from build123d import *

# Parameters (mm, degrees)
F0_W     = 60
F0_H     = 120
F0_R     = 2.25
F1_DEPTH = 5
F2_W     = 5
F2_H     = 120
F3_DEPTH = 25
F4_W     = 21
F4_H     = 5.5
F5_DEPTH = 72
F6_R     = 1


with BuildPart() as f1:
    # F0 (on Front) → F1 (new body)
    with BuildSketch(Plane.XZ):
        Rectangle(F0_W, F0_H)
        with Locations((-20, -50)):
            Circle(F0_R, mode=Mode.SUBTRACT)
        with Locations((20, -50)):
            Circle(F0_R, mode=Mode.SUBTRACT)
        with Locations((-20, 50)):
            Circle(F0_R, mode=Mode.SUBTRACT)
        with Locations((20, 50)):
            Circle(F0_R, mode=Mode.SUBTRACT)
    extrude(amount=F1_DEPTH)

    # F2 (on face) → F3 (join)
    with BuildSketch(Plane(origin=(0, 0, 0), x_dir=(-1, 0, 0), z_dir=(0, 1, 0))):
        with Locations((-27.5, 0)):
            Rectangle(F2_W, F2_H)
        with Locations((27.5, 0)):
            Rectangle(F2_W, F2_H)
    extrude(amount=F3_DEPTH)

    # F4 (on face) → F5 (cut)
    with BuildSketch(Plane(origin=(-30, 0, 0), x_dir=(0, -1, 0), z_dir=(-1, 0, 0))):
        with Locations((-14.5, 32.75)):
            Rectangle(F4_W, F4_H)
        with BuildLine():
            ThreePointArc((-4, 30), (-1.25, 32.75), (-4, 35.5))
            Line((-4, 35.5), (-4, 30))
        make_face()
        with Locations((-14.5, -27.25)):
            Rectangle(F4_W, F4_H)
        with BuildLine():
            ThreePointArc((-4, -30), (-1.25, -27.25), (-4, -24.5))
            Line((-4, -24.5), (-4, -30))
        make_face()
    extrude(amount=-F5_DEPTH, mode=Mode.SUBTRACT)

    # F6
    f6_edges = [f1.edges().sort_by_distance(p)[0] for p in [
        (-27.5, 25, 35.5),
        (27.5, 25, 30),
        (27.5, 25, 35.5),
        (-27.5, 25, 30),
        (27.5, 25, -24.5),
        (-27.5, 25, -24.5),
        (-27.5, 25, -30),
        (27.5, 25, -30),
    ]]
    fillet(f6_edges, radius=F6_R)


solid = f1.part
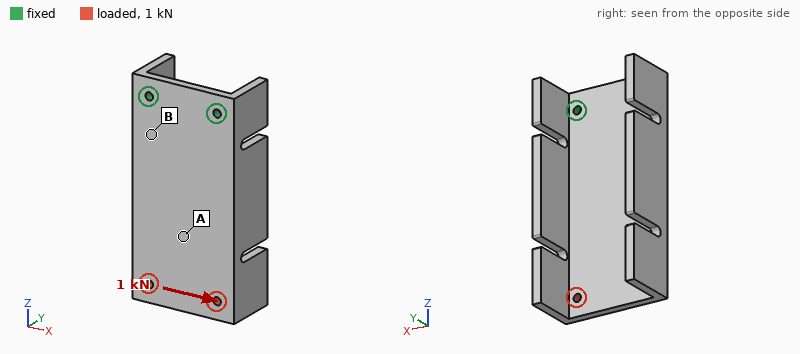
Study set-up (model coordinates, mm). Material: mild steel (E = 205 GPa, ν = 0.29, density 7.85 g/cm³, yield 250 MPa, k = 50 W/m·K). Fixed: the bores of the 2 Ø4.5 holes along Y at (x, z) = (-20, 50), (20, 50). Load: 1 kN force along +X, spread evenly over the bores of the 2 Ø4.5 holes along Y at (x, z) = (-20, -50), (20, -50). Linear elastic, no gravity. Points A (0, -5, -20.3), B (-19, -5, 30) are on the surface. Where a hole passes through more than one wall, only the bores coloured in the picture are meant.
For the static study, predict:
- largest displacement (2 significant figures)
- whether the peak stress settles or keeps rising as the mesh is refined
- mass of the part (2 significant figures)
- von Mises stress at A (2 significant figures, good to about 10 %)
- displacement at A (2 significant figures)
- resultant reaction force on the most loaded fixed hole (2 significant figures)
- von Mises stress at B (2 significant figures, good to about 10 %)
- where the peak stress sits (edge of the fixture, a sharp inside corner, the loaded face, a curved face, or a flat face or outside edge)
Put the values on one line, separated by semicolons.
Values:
29 µm; keeps rising; 500 g; 5.5 MPa; 14 µm; 2.4 kN; 16 MPa; edge of the fixture
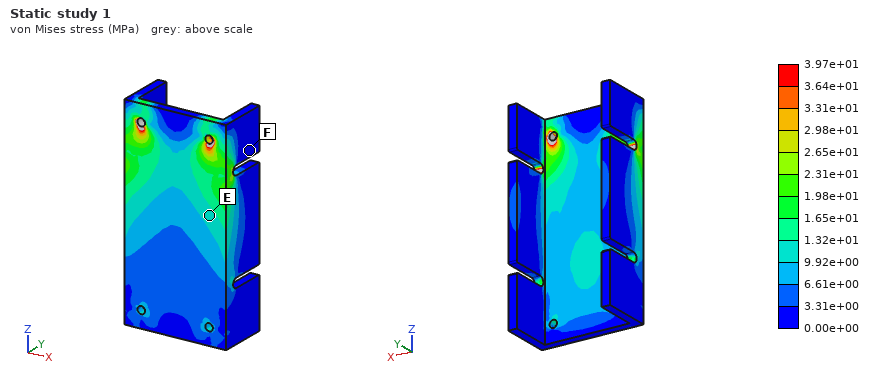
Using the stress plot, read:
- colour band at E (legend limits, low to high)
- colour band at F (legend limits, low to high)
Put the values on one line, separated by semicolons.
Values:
9.92e+00 to 1.32e+01 MPa; 0.00e+00 to 3.31e+00 MPa
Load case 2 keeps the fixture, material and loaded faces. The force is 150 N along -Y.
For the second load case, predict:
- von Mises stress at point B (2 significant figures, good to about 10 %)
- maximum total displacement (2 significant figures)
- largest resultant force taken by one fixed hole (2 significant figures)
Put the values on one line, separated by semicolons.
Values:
33 MPa; 0.21 mm; 110 N
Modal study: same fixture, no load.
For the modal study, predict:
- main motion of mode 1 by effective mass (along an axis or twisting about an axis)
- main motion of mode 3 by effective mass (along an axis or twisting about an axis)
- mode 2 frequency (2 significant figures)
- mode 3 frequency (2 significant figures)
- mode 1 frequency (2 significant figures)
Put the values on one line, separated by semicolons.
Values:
along Y; along X; 850 Hz; 2400 Hz; 360 Hz
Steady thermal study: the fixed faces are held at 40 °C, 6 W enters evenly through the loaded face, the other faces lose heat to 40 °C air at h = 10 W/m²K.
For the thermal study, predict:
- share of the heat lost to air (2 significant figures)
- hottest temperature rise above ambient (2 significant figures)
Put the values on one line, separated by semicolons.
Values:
48 %; 24 K
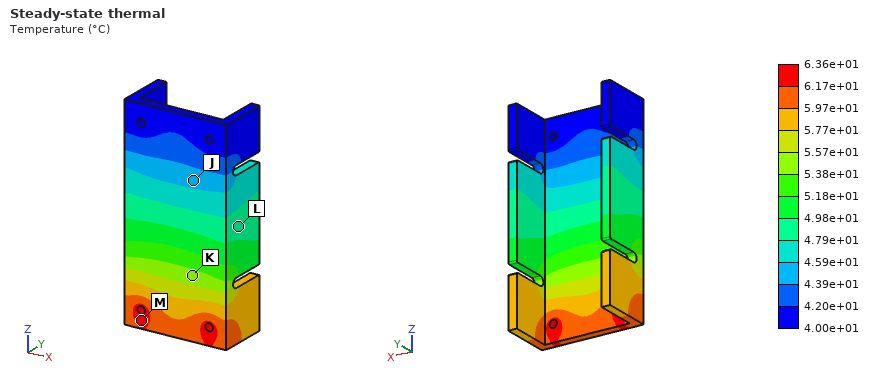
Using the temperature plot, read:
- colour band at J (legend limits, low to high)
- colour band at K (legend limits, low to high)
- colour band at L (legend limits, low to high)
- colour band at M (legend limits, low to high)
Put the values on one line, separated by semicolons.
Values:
4.39e+01 to 4.59e+01 °C; 5.38e+01 to 5.57e+01 °C; 4.79e+01 to 4.98e+01 °C; 6.17e+01 to 6.36e+01 °C
